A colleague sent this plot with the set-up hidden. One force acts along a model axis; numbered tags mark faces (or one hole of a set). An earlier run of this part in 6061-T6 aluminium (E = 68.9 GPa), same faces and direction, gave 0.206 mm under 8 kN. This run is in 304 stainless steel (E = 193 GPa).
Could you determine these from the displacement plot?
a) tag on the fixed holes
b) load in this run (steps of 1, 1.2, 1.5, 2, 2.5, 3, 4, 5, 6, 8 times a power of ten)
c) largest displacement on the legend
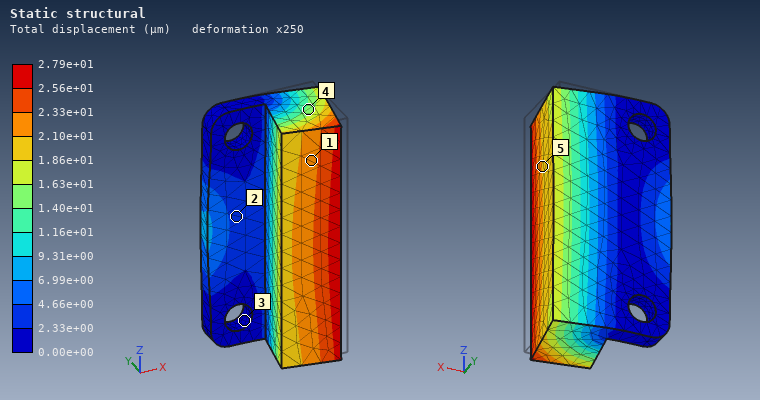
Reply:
3
3 kN
2.79e+01 µm
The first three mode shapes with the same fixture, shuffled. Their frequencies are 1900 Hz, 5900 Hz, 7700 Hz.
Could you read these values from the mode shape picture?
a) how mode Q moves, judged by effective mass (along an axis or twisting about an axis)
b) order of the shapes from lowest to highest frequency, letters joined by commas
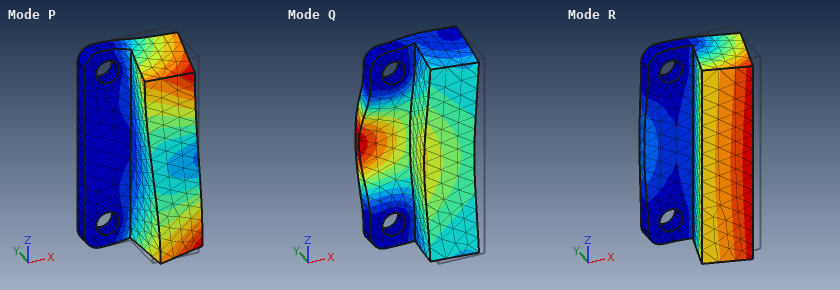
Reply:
along Y
R, P, Q
